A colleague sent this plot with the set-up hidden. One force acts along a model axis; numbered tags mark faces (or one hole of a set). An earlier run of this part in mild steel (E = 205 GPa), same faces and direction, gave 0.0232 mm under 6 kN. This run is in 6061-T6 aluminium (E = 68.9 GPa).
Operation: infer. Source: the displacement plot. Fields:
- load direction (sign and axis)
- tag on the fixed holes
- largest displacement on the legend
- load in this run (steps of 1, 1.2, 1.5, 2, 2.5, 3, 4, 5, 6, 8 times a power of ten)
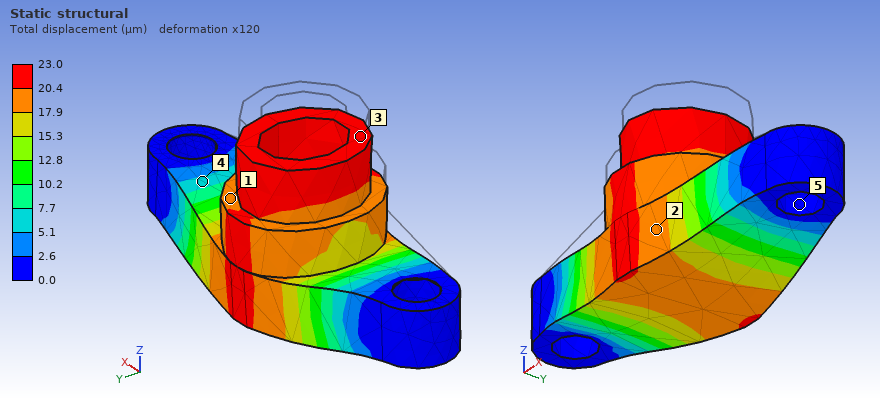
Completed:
-Z
5
23.0 µm
2 kN
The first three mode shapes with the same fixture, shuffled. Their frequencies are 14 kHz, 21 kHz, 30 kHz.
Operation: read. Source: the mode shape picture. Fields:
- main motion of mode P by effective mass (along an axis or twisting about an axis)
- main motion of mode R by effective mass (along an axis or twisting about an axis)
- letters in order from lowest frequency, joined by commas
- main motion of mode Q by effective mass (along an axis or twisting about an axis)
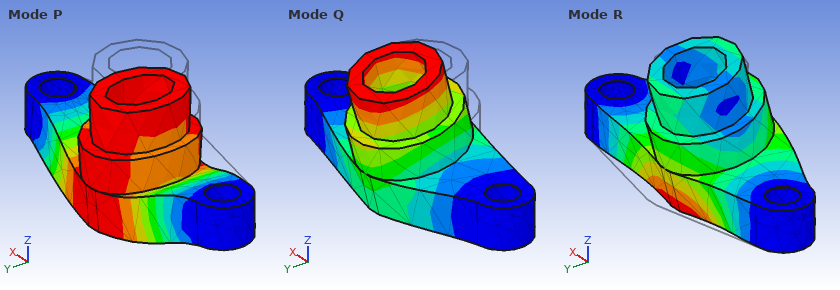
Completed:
along Z
along Y
Q, P, R
along Y
